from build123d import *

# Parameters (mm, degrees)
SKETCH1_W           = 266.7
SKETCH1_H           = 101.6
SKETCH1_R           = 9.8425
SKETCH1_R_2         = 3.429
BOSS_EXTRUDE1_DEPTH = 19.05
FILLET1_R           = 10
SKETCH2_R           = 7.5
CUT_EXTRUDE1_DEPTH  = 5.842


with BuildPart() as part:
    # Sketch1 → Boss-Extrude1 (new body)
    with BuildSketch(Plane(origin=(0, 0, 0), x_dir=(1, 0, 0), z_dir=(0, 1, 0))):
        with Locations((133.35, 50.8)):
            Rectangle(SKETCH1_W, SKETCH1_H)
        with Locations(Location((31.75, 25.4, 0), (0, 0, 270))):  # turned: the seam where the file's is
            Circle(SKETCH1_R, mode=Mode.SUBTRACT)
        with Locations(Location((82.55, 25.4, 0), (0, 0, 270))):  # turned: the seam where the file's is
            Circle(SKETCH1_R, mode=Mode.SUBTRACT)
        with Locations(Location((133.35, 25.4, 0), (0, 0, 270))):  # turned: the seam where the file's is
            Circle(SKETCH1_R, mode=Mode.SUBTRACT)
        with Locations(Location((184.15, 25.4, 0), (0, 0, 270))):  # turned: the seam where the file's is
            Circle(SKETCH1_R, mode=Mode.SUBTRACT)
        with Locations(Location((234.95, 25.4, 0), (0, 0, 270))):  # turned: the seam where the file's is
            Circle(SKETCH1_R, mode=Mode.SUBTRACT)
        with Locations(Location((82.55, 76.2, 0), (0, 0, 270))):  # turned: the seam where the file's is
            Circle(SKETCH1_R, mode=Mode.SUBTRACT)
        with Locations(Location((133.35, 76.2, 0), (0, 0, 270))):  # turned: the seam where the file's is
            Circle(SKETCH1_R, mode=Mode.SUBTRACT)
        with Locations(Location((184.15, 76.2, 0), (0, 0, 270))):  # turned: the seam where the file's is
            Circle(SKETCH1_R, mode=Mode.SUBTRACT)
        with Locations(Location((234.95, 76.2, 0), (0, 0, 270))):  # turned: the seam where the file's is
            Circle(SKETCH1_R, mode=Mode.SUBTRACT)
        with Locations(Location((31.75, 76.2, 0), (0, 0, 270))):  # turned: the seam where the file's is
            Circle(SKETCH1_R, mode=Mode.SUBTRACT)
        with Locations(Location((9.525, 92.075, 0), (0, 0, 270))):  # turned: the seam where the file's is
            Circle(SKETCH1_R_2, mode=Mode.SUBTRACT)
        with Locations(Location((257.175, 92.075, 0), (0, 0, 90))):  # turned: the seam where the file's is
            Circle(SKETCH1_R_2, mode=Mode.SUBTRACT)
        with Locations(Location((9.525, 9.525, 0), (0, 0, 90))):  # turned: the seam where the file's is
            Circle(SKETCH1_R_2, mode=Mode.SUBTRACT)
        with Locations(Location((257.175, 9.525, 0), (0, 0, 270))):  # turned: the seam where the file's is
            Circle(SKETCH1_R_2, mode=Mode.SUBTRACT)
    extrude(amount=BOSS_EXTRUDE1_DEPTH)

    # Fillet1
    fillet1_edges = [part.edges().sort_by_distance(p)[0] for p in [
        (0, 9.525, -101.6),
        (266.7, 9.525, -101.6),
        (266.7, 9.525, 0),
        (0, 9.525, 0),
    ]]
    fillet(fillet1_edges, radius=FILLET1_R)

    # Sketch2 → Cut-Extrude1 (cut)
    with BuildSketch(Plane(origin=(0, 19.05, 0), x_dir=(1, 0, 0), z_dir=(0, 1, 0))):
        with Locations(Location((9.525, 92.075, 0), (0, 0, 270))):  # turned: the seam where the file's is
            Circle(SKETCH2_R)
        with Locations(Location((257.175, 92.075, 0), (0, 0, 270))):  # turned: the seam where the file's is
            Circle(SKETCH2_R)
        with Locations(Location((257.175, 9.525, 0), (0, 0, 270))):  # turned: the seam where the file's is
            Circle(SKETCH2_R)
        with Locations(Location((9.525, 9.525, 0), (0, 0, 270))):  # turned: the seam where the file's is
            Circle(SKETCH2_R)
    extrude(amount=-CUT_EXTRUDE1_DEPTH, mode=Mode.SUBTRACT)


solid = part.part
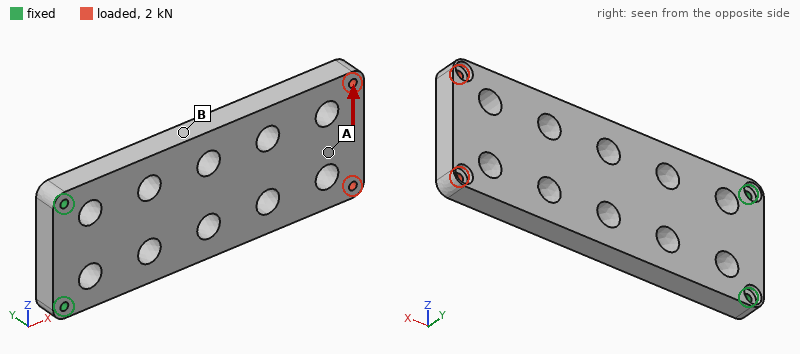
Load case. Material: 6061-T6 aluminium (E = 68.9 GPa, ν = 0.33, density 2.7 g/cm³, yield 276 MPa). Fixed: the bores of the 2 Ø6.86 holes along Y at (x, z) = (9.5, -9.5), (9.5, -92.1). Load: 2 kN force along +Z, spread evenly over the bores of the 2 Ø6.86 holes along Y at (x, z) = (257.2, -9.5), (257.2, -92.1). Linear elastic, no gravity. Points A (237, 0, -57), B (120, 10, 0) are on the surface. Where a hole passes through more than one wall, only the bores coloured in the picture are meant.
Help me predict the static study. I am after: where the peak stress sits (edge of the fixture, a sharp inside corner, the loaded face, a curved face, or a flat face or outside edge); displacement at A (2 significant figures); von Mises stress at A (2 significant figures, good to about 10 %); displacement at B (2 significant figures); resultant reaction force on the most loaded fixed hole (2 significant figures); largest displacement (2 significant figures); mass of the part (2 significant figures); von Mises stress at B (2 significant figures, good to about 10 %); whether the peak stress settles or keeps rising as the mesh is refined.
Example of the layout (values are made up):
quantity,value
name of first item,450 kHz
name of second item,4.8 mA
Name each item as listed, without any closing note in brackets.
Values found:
quantity,value
where the peak stress sits,edge of the fixture
displacement at A,0.13 mm
von Mises stress at A,5.5 MPa
displacement at B,0.053 mm
resultant reaction force on the most loaded fixed hole,5.9 kN
largest displacement,0.16 mm
mass of the part,1.2 kg
von Mises stress at B,12 MPa
whether the peak stress settles or keeps rising as the mesh is refined,keeps rising
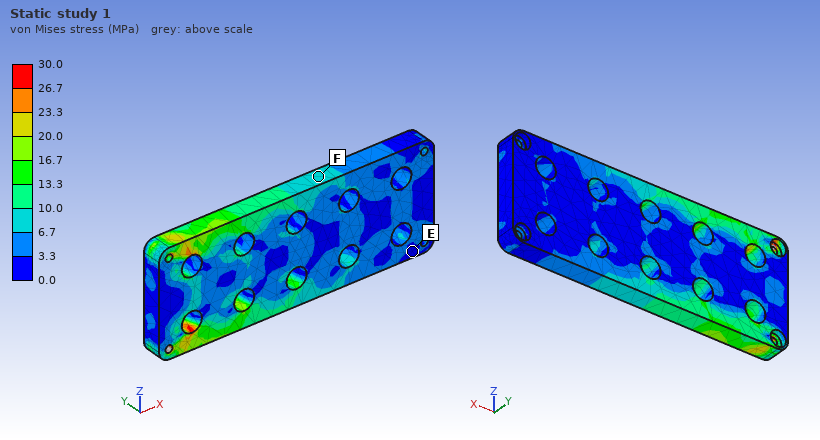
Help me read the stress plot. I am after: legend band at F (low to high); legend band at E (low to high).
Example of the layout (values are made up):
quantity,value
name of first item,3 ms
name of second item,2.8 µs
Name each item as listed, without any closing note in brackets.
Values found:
quantity,value
legend band at F,6.7 to 10.0 MPa
legend band at E,0.0 to 3.3 MPa
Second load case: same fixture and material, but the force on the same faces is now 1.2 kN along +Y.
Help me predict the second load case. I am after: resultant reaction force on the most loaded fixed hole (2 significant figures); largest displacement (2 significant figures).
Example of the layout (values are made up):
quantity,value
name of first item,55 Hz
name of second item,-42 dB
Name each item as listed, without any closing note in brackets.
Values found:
quantity,value
resultant reaction force on the most loaded fixed hole,610 N
largest displacement,2.9 mm
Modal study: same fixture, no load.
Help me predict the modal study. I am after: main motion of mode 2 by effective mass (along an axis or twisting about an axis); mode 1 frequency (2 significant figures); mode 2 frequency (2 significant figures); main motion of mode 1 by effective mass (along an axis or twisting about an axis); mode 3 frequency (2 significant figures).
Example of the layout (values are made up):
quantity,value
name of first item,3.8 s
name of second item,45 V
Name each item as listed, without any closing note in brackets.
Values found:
quantity,value
main motion of mode 2 by effective mass,along Z
mode 1 frequency,180 Hz
mode 2 frequency,980 Hz
main motion of mode 1 by effective mass,along Y
mode 3 frequency,1100 Hz
